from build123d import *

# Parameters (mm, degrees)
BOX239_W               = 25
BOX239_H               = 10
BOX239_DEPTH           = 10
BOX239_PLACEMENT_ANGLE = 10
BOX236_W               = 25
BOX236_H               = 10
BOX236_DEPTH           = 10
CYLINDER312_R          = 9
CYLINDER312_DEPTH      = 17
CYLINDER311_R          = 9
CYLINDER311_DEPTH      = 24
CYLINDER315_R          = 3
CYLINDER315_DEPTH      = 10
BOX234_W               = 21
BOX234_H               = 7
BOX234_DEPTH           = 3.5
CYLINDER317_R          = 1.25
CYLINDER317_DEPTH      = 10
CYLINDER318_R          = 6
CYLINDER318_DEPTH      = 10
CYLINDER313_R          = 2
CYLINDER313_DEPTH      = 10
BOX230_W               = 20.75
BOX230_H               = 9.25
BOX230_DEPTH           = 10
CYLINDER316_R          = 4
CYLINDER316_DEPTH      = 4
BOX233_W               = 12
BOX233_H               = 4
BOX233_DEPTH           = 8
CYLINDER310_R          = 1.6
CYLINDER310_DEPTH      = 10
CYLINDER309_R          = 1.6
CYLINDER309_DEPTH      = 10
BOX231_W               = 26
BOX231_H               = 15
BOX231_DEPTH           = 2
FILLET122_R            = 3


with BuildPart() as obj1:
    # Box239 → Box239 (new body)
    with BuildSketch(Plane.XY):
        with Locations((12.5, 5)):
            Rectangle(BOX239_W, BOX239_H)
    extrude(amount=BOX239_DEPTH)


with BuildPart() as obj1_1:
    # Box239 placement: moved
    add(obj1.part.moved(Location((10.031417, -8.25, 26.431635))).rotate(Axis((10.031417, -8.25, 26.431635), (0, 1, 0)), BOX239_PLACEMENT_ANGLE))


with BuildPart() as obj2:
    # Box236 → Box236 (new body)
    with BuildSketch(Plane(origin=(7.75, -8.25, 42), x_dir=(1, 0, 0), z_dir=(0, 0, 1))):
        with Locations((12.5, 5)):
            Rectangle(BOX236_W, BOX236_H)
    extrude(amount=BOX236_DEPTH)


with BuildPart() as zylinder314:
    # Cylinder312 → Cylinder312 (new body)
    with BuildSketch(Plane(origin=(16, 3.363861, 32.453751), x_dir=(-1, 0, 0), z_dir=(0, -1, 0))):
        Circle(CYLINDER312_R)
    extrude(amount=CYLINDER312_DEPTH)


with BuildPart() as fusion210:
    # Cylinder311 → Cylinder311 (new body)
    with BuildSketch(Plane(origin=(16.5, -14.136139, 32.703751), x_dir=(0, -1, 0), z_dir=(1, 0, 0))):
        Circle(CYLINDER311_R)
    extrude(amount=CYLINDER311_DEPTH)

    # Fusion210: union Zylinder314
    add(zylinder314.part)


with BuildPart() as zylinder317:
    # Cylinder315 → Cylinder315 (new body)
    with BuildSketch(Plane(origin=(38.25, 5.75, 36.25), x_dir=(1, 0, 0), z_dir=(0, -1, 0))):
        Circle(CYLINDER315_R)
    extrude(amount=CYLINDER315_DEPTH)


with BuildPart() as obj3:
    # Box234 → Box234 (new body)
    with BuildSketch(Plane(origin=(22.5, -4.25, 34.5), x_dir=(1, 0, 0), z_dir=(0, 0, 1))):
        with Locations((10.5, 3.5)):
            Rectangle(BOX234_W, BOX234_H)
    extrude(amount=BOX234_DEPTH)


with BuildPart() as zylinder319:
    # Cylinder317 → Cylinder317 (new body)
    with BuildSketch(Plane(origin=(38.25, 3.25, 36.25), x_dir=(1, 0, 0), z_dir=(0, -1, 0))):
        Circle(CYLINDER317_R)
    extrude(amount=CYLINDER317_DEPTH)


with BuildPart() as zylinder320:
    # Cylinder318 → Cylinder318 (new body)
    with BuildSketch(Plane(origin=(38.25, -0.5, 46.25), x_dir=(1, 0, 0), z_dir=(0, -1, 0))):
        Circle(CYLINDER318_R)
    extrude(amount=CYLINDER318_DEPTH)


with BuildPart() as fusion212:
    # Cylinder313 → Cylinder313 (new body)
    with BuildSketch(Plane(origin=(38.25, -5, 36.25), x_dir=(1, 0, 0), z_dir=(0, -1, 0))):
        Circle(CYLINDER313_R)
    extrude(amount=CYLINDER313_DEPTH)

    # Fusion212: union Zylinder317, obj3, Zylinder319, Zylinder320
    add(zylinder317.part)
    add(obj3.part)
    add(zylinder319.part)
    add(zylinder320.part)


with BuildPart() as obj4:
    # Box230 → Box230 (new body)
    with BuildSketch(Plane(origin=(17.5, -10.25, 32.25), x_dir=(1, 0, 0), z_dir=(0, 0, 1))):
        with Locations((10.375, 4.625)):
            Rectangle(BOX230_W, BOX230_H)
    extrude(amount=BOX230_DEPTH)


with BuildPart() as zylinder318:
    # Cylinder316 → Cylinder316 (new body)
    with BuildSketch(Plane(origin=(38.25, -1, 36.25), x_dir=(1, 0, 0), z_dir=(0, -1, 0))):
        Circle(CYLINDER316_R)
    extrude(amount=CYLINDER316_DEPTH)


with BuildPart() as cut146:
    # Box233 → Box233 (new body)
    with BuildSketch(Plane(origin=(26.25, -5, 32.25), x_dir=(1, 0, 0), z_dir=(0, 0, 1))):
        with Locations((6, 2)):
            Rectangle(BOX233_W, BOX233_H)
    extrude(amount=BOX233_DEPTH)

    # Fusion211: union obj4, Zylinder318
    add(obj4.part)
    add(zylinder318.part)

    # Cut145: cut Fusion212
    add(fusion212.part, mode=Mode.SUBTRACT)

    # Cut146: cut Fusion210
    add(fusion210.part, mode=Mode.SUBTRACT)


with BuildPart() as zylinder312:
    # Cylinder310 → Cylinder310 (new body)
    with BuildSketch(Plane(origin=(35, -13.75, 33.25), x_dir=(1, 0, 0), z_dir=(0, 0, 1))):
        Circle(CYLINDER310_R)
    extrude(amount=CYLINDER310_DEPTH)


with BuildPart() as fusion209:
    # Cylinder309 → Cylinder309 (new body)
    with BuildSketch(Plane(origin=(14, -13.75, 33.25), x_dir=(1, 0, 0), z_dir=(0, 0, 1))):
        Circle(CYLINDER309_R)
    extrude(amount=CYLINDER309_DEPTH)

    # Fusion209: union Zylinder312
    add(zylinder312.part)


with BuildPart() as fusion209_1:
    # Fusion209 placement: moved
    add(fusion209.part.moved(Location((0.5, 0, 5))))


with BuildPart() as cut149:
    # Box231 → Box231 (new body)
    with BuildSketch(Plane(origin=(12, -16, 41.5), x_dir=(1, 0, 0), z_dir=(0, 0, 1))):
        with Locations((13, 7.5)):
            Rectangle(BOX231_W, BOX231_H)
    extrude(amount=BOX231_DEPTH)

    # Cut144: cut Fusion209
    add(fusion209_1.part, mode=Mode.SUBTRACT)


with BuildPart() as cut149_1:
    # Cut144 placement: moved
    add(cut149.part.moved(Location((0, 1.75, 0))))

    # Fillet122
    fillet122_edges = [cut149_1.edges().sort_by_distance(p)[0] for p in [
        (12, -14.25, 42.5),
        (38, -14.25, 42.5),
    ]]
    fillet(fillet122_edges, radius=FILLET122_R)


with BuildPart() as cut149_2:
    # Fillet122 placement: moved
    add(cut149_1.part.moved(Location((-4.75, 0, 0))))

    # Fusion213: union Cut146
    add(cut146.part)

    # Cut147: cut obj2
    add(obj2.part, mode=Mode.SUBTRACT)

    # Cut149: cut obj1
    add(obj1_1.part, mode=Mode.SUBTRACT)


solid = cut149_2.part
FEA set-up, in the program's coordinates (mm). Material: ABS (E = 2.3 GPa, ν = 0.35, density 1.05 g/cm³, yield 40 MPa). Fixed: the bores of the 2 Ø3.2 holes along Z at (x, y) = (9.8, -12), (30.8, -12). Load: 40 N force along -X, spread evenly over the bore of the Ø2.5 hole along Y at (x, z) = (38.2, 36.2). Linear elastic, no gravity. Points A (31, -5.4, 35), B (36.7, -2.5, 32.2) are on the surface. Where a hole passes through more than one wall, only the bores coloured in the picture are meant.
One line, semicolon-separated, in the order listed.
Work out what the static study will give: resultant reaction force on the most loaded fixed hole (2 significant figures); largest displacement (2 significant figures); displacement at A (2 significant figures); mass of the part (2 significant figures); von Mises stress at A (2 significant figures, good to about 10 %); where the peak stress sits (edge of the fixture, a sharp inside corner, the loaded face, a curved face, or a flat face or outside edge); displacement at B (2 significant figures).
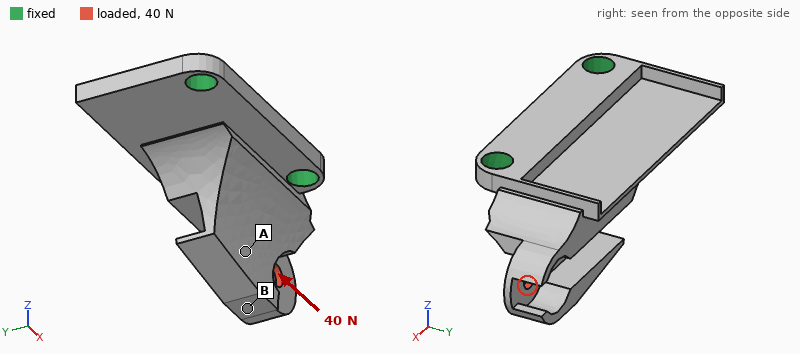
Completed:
25 N; 0.17 mm; 0.080 mm; 1.1 g; 3.7 MPa; edge of the fixture; 0.13 mm
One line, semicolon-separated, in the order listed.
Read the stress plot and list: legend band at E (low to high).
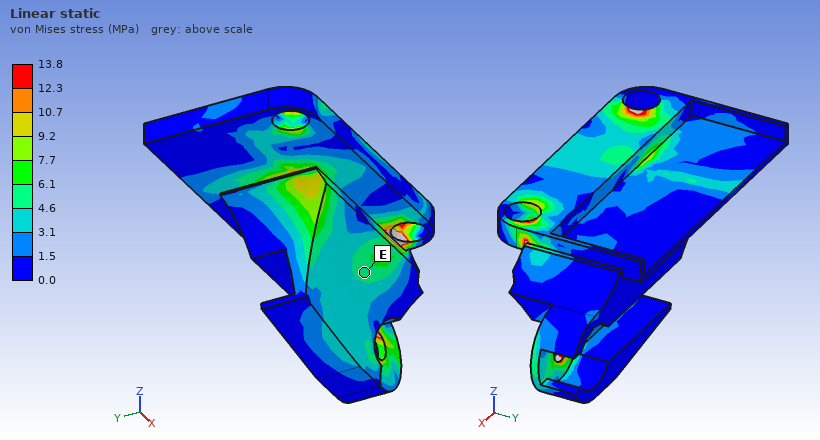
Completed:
4.6 to 6.1 MPa
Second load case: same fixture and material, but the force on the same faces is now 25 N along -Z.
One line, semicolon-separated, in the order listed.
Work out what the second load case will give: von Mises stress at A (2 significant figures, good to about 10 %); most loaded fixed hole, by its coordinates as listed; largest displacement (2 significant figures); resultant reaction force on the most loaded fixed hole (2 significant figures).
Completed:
3.2 MPa; (30.8, -12); 0.48 mm; 32 N
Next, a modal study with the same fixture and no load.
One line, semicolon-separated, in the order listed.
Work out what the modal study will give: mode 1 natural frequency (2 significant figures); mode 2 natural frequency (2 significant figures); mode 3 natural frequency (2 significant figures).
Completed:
1900 Hz; 3400 Hz; 4000 Hz
